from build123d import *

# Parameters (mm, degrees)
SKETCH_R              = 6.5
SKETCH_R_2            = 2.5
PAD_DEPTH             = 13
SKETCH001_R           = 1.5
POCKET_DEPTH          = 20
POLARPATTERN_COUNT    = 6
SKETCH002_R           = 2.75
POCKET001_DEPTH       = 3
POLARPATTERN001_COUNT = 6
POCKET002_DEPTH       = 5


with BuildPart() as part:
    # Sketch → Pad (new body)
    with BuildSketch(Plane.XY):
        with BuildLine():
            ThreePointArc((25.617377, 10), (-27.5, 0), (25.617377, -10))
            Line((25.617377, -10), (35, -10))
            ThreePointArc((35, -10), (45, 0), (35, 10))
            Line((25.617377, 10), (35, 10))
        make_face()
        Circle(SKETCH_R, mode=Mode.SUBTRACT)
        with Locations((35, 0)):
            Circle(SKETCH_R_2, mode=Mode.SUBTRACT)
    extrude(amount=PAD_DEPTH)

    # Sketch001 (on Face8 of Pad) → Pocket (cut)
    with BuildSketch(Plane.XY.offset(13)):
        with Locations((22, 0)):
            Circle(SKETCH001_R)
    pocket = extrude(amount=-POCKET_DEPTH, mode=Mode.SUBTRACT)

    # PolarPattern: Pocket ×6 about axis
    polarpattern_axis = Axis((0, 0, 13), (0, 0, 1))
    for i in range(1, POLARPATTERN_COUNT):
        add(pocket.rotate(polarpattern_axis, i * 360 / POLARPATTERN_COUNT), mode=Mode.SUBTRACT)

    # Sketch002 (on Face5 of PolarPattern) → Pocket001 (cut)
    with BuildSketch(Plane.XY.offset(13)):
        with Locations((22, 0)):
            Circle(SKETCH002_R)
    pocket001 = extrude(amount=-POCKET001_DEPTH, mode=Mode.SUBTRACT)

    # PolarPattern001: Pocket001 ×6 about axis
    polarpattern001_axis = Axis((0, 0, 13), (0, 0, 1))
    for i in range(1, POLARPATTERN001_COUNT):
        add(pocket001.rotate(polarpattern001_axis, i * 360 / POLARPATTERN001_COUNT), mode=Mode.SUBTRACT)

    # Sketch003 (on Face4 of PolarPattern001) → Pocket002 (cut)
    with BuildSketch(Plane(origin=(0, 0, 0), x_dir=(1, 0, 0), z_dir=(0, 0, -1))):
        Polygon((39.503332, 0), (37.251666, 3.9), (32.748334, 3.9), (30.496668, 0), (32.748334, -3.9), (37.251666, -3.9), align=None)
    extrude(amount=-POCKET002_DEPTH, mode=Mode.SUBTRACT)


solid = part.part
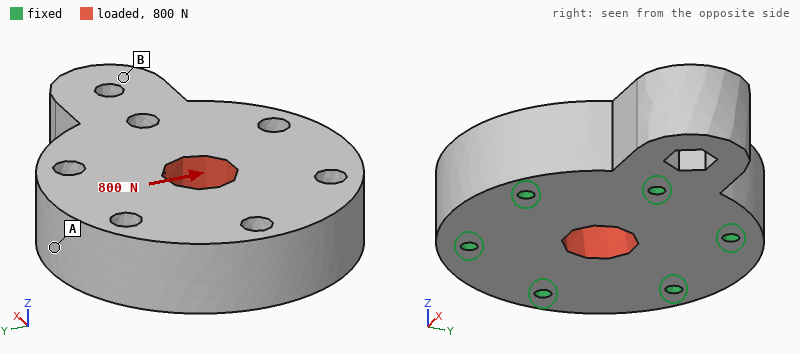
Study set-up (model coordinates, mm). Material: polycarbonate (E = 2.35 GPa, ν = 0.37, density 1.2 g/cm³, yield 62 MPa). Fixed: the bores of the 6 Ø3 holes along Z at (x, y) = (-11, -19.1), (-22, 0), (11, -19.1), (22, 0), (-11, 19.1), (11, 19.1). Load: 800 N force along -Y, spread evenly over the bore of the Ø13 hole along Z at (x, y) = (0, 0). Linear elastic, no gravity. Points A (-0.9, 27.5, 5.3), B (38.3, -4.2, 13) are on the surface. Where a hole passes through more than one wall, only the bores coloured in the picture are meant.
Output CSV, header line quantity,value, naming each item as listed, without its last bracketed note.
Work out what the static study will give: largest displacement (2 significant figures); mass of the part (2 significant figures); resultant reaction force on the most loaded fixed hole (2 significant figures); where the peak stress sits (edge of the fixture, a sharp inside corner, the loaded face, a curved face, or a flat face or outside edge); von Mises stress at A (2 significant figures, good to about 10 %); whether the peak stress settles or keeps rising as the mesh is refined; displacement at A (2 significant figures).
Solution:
quantity,value
largest displacement,12 µm
mass of the part,38 g
resultant reaction force on the most loaded fixed hole,170 N
where the peak stress sits,edge of the fixture
von Mises stress at A,0.71 MPa
whether the peak stress settles or keeps rising as the mesh is refined,keeps rising
displacement at A,4.8 µm
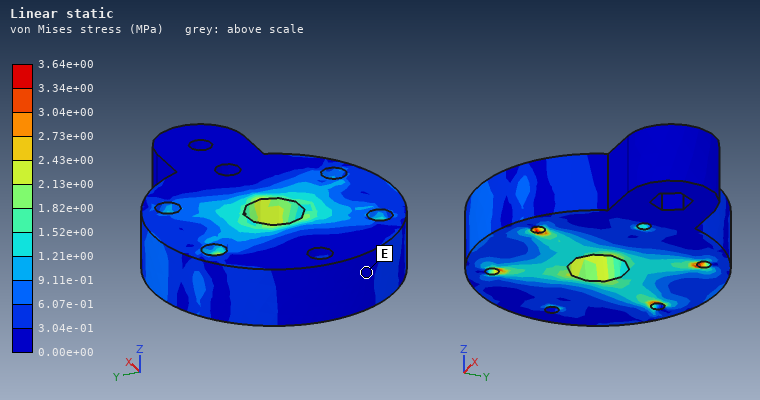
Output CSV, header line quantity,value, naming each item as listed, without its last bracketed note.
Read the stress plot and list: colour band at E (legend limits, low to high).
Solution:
quantity,value
colour band at E,0.00e+00 to 3.04e-01 MPa
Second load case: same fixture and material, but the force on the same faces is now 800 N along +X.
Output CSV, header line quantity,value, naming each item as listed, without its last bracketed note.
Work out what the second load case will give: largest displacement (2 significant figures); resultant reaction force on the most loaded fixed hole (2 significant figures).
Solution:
quantity,value
largest displacement,12 µm
resultant reaction force on the most loaded fixed hole,210 N
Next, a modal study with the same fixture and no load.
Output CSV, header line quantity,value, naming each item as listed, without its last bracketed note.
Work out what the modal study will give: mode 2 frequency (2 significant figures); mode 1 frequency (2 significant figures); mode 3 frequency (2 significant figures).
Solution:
quantity,value
mode 2 frequency,5900 Hz
mode 1 frequency,4200 Hz
mode 3 frequency,7800 Hz
